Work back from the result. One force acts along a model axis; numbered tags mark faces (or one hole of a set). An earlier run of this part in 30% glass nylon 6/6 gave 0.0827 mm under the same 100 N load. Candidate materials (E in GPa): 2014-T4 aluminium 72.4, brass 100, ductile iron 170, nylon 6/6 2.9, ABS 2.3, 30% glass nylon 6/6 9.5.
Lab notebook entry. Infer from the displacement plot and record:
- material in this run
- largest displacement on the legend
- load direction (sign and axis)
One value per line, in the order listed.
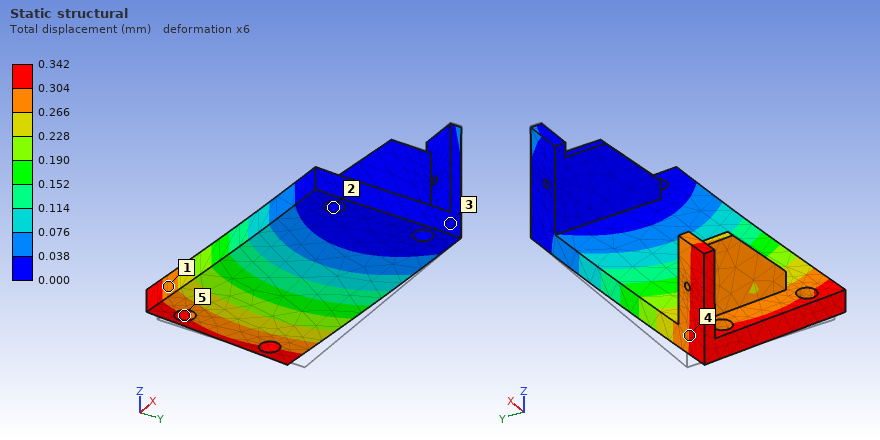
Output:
ABS
0.342 mm
-Y
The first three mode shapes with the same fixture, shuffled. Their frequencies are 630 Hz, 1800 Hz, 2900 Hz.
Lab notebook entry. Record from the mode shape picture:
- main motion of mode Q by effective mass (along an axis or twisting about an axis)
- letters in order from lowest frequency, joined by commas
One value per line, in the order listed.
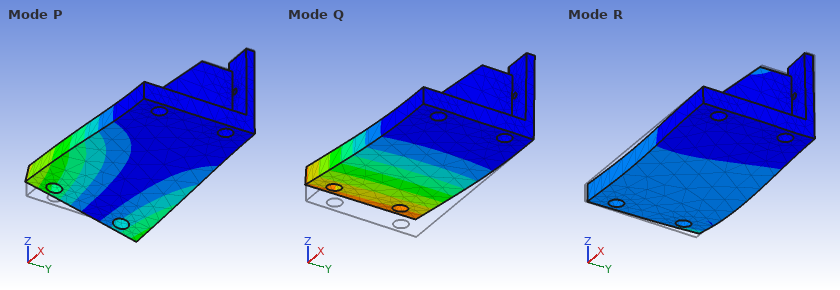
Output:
along Z
Q, P, R
